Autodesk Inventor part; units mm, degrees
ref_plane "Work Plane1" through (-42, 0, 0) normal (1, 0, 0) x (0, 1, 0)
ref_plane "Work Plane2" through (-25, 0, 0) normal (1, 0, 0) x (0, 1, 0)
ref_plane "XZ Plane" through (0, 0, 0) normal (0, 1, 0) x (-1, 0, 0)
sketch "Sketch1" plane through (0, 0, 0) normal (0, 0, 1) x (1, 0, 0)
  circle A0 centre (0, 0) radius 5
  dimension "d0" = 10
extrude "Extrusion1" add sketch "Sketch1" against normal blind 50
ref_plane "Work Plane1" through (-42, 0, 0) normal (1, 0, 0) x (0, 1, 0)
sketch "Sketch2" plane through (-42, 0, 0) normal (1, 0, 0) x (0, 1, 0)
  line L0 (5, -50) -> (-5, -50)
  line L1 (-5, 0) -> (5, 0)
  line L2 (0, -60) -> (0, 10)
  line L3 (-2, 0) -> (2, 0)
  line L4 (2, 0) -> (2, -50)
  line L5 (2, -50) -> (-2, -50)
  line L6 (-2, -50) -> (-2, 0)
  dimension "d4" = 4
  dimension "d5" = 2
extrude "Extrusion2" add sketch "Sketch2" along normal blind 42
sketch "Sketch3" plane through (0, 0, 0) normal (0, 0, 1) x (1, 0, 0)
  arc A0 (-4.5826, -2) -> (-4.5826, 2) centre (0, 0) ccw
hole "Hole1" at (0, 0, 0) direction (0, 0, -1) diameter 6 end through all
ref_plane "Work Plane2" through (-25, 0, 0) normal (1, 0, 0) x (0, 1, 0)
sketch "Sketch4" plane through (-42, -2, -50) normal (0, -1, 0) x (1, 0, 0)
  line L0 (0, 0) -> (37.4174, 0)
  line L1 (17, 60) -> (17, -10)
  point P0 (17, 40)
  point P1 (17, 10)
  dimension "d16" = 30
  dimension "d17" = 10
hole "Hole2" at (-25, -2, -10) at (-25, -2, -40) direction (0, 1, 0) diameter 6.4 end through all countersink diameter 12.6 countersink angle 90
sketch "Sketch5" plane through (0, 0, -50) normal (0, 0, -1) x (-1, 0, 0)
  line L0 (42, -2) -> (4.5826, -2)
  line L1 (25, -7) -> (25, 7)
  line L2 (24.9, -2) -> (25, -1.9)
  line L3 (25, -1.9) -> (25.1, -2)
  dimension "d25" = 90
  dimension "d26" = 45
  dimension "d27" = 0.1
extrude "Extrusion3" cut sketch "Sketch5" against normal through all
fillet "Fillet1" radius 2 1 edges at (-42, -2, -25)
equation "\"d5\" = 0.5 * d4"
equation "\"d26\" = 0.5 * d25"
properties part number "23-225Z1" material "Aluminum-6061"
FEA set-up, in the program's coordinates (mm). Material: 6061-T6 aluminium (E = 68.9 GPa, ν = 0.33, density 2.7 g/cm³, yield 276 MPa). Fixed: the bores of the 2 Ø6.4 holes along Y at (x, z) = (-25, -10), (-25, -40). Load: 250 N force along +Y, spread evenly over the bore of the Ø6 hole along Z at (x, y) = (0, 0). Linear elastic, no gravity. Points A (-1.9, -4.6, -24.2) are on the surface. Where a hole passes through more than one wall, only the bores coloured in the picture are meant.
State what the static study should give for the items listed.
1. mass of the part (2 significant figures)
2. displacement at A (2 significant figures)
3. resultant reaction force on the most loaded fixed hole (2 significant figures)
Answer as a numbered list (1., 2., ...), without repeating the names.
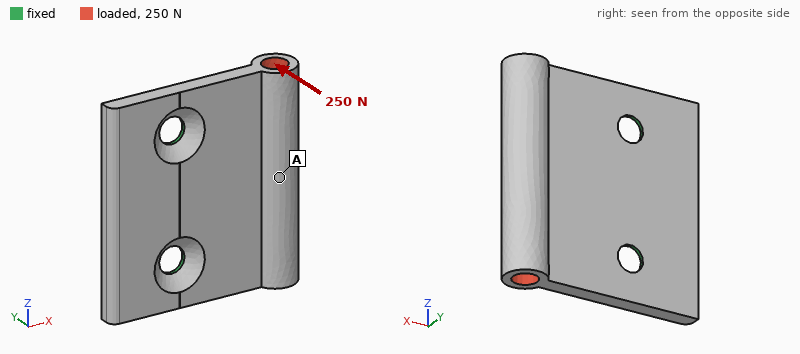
1. 25 g
2. 0.14 mm
3. 150 N
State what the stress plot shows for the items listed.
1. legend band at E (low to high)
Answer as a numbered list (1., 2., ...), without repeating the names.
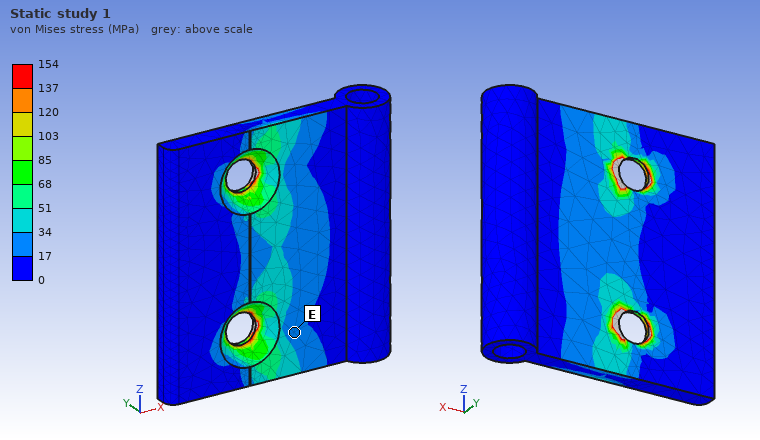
1. 17 to 34 MPa
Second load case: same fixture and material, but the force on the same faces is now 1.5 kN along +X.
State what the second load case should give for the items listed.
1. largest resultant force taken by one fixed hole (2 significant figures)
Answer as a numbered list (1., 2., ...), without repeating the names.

1. 750 N
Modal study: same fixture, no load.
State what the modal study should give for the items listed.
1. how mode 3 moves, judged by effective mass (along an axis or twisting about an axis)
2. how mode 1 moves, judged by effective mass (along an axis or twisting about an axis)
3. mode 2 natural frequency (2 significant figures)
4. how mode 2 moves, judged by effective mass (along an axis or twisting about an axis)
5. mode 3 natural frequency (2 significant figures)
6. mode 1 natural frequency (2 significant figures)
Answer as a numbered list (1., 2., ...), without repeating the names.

1. along Y
2. along Y
3. 5400 Hz
4. twisting about X
5. 7700 Hz
6. 2200 Hz
